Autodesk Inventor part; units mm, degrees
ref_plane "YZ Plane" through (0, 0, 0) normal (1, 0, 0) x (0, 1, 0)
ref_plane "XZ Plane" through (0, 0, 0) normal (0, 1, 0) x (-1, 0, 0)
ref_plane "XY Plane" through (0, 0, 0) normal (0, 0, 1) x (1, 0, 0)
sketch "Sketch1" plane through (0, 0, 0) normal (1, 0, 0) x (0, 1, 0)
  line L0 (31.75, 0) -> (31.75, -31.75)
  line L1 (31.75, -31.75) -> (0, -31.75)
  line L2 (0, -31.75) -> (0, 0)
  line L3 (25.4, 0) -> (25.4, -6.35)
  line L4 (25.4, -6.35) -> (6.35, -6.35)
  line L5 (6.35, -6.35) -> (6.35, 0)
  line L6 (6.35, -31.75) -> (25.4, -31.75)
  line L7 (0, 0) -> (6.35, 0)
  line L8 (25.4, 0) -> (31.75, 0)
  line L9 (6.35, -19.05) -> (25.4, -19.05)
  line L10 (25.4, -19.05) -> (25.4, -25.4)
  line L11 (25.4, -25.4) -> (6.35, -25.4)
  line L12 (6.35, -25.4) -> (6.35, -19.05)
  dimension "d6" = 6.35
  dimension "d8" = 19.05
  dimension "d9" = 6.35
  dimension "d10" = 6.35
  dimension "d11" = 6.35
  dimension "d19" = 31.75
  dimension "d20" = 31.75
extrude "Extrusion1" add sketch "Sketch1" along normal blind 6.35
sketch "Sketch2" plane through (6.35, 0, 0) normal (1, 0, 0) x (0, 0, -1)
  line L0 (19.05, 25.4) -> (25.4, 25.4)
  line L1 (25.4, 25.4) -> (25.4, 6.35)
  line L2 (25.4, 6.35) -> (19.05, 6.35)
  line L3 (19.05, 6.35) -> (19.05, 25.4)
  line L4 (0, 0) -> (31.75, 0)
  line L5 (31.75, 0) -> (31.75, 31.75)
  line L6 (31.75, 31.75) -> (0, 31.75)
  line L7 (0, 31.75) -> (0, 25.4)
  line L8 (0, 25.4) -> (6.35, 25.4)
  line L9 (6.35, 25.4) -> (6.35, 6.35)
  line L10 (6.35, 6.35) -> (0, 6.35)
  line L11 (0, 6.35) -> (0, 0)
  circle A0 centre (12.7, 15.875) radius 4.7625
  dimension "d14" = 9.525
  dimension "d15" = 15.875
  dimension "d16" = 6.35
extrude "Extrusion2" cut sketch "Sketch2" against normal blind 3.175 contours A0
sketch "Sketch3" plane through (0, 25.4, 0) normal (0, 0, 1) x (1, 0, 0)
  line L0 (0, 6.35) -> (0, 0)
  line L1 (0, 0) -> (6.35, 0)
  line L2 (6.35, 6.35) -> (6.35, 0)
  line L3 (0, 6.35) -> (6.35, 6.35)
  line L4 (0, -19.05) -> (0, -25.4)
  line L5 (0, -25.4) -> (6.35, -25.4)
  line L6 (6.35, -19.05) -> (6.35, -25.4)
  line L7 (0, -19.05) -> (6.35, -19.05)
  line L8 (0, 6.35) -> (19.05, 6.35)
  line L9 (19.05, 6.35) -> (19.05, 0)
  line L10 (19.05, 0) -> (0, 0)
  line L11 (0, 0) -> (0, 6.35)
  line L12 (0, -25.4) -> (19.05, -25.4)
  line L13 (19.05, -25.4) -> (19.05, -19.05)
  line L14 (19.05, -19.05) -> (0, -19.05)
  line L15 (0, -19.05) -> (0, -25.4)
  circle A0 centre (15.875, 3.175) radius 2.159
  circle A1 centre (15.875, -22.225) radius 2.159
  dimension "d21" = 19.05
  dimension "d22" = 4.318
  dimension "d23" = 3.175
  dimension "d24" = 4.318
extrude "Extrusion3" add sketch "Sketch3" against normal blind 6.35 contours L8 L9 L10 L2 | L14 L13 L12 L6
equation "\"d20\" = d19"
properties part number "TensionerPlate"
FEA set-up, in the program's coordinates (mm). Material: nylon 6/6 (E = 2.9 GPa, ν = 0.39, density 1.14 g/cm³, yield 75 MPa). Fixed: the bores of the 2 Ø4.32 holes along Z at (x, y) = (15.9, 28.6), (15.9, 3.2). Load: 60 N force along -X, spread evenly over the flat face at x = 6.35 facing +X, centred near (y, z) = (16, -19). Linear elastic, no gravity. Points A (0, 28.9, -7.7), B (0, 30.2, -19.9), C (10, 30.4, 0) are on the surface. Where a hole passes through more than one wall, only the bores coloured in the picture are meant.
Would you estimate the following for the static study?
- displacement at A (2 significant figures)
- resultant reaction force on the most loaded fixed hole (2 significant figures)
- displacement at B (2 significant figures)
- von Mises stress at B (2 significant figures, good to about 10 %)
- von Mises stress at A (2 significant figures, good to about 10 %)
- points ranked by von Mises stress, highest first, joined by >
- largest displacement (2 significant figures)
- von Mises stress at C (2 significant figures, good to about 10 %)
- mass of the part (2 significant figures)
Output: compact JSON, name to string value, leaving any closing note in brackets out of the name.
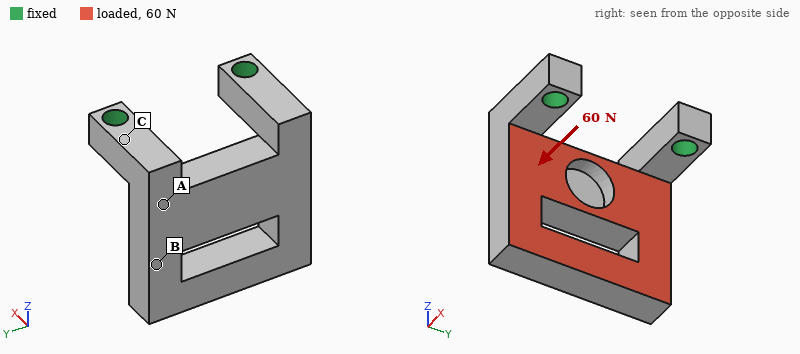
{"displacement at A": "0.14 mm", "resultant reaction force on the most loaded fixed hole": "30 N", "displacement at B": "0.32 mm", "von Mises stress at B": "2.1 MPa", "von Mises stress at A": "6.8 MPa", "points ranked by von Mises stress, highest first, joined by >": "C > A > B", "largest displacement": "0.57 mm", "von Mises stress at C": "11 MPa", "mass of the part": "6.2 g"}
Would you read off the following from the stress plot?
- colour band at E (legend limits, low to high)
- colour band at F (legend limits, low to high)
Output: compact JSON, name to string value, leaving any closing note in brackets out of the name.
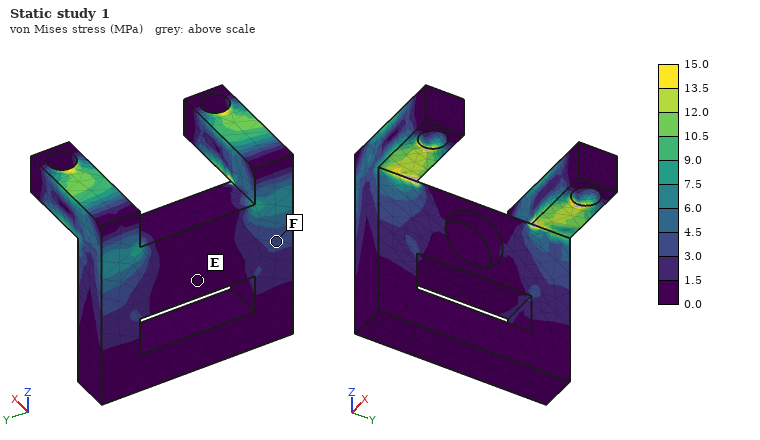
{"colour band at E": "0.0 to 1.5 MPa", "colour band at F": "3.0 to 4.5 MPa"}
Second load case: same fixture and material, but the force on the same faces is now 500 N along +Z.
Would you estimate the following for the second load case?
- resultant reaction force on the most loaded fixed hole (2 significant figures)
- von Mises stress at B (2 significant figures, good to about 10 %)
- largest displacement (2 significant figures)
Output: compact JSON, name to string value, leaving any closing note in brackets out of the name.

{"resultant reaction force on the most loaded fixed hole": "250 N", "von Mises stress at B": "5.4 MPa", "largest displacement": "0.36 mm"}
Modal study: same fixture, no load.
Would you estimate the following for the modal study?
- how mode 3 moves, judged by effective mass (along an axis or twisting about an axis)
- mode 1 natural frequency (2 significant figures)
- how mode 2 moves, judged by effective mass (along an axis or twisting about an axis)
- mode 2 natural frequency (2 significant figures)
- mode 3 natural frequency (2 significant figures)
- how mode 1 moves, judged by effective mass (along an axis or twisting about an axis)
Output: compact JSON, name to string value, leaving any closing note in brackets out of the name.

{"how mode 3 moves, judged by effective mass": "along Y", "mode 1 natural frequency": "910 Hz", "how mode 2 moves, judged by effective mass": "along Y", "mode 2 natural frequency": "1800 Hz", "mode 3 natural frequency": "2800 Hz", "how mode 1 moves, judged by effective mass": "along X"}
